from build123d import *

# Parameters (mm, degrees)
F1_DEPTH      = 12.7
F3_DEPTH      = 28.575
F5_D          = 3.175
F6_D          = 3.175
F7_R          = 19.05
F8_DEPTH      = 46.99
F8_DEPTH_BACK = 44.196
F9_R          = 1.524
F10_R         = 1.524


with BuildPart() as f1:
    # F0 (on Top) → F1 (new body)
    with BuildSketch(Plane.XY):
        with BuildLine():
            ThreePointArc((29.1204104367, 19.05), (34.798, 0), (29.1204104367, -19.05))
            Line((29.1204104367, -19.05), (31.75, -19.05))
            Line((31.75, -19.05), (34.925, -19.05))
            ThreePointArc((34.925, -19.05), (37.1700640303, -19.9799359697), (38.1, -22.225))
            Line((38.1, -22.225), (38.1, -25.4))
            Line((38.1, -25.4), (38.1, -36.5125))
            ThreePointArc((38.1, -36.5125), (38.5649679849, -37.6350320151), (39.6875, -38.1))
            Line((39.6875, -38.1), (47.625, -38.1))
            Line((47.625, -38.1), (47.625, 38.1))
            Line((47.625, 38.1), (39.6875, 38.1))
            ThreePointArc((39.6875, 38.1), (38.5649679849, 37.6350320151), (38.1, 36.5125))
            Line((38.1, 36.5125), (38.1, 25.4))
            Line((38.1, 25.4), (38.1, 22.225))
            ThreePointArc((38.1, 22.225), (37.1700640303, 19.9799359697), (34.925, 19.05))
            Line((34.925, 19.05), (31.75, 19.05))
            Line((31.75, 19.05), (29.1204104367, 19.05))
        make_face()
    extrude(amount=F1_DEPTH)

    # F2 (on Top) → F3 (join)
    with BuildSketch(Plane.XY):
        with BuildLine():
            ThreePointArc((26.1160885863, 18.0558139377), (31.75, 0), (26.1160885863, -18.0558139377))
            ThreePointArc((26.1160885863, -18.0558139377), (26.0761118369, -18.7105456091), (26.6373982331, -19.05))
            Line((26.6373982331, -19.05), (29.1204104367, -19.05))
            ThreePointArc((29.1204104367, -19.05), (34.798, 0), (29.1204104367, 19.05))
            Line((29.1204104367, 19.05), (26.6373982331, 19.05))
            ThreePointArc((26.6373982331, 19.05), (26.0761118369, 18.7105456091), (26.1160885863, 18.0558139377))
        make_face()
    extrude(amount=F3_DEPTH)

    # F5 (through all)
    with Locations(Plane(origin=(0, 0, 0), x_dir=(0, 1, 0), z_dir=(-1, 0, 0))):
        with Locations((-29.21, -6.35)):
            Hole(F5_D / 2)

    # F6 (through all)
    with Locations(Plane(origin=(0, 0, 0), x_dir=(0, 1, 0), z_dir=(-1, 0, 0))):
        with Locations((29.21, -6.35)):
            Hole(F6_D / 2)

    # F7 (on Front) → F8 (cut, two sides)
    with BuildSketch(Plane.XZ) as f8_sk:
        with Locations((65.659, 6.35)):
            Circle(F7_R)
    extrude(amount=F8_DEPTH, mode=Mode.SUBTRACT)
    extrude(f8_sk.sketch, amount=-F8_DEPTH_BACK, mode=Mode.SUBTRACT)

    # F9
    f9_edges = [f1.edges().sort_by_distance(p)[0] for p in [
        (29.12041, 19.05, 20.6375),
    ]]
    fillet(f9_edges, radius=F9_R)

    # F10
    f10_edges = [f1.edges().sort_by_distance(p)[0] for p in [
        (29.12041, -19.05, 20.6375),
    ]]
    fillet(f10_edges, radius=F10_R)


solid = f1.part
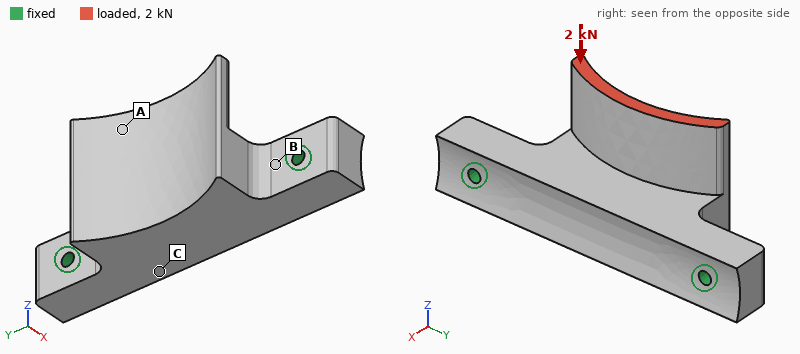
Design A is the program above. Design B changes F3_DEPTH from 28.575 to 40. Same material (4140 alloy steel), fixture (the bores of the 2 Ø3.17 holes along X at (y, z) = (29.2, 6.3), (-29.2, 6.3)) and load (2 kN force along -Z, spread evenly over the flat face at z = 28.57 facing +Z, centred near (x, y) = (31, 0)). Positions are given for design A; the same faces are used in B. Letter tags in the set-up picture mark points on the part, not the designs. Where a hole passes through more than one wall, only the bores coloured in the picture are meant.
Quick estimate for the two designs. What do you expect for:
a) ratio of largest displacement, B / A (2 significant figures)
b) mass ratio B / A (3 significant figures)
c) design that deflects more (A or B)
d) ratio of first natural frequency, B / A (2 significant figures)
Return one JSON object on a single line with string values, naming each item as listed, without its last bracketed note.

{"ratio of largest displacement, B / A": "1.2", "mass ratio B / A": "1.10", "design that deflects more": "B", "ratio of first natural frequency, B / A": "0.59"}
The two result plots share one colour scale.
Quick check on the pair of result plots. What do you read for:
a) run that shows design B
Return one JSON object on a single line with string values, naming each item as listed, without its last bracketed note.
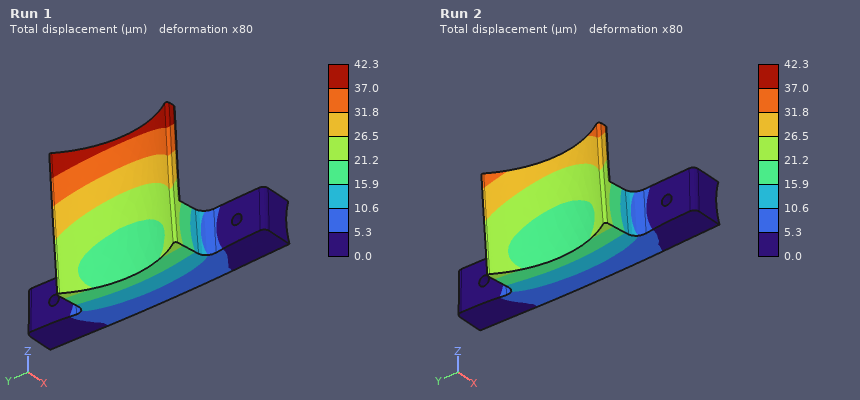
{"run that shows design B": "Run 1"}
